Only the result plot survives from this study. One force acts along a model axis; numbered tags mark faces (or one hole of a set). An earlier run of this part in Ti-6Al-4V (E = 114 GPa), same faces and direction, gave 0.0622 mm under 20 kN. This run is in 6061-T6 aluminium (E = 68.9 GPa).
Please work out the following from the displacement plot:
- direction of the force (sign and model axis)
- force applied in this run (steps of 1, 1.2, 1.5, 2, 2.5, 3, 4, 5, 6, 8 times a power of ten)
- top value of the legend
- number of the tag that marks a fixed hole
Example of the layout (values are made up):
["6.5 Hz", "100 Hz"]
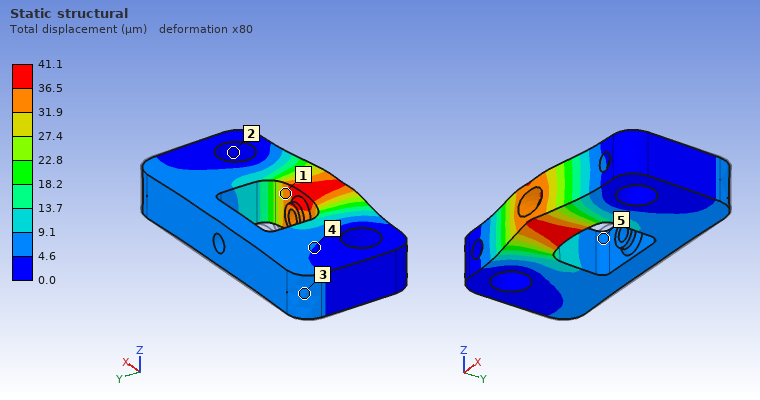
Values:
["-Y", "8 kN", "41.1 µm", "2"]
